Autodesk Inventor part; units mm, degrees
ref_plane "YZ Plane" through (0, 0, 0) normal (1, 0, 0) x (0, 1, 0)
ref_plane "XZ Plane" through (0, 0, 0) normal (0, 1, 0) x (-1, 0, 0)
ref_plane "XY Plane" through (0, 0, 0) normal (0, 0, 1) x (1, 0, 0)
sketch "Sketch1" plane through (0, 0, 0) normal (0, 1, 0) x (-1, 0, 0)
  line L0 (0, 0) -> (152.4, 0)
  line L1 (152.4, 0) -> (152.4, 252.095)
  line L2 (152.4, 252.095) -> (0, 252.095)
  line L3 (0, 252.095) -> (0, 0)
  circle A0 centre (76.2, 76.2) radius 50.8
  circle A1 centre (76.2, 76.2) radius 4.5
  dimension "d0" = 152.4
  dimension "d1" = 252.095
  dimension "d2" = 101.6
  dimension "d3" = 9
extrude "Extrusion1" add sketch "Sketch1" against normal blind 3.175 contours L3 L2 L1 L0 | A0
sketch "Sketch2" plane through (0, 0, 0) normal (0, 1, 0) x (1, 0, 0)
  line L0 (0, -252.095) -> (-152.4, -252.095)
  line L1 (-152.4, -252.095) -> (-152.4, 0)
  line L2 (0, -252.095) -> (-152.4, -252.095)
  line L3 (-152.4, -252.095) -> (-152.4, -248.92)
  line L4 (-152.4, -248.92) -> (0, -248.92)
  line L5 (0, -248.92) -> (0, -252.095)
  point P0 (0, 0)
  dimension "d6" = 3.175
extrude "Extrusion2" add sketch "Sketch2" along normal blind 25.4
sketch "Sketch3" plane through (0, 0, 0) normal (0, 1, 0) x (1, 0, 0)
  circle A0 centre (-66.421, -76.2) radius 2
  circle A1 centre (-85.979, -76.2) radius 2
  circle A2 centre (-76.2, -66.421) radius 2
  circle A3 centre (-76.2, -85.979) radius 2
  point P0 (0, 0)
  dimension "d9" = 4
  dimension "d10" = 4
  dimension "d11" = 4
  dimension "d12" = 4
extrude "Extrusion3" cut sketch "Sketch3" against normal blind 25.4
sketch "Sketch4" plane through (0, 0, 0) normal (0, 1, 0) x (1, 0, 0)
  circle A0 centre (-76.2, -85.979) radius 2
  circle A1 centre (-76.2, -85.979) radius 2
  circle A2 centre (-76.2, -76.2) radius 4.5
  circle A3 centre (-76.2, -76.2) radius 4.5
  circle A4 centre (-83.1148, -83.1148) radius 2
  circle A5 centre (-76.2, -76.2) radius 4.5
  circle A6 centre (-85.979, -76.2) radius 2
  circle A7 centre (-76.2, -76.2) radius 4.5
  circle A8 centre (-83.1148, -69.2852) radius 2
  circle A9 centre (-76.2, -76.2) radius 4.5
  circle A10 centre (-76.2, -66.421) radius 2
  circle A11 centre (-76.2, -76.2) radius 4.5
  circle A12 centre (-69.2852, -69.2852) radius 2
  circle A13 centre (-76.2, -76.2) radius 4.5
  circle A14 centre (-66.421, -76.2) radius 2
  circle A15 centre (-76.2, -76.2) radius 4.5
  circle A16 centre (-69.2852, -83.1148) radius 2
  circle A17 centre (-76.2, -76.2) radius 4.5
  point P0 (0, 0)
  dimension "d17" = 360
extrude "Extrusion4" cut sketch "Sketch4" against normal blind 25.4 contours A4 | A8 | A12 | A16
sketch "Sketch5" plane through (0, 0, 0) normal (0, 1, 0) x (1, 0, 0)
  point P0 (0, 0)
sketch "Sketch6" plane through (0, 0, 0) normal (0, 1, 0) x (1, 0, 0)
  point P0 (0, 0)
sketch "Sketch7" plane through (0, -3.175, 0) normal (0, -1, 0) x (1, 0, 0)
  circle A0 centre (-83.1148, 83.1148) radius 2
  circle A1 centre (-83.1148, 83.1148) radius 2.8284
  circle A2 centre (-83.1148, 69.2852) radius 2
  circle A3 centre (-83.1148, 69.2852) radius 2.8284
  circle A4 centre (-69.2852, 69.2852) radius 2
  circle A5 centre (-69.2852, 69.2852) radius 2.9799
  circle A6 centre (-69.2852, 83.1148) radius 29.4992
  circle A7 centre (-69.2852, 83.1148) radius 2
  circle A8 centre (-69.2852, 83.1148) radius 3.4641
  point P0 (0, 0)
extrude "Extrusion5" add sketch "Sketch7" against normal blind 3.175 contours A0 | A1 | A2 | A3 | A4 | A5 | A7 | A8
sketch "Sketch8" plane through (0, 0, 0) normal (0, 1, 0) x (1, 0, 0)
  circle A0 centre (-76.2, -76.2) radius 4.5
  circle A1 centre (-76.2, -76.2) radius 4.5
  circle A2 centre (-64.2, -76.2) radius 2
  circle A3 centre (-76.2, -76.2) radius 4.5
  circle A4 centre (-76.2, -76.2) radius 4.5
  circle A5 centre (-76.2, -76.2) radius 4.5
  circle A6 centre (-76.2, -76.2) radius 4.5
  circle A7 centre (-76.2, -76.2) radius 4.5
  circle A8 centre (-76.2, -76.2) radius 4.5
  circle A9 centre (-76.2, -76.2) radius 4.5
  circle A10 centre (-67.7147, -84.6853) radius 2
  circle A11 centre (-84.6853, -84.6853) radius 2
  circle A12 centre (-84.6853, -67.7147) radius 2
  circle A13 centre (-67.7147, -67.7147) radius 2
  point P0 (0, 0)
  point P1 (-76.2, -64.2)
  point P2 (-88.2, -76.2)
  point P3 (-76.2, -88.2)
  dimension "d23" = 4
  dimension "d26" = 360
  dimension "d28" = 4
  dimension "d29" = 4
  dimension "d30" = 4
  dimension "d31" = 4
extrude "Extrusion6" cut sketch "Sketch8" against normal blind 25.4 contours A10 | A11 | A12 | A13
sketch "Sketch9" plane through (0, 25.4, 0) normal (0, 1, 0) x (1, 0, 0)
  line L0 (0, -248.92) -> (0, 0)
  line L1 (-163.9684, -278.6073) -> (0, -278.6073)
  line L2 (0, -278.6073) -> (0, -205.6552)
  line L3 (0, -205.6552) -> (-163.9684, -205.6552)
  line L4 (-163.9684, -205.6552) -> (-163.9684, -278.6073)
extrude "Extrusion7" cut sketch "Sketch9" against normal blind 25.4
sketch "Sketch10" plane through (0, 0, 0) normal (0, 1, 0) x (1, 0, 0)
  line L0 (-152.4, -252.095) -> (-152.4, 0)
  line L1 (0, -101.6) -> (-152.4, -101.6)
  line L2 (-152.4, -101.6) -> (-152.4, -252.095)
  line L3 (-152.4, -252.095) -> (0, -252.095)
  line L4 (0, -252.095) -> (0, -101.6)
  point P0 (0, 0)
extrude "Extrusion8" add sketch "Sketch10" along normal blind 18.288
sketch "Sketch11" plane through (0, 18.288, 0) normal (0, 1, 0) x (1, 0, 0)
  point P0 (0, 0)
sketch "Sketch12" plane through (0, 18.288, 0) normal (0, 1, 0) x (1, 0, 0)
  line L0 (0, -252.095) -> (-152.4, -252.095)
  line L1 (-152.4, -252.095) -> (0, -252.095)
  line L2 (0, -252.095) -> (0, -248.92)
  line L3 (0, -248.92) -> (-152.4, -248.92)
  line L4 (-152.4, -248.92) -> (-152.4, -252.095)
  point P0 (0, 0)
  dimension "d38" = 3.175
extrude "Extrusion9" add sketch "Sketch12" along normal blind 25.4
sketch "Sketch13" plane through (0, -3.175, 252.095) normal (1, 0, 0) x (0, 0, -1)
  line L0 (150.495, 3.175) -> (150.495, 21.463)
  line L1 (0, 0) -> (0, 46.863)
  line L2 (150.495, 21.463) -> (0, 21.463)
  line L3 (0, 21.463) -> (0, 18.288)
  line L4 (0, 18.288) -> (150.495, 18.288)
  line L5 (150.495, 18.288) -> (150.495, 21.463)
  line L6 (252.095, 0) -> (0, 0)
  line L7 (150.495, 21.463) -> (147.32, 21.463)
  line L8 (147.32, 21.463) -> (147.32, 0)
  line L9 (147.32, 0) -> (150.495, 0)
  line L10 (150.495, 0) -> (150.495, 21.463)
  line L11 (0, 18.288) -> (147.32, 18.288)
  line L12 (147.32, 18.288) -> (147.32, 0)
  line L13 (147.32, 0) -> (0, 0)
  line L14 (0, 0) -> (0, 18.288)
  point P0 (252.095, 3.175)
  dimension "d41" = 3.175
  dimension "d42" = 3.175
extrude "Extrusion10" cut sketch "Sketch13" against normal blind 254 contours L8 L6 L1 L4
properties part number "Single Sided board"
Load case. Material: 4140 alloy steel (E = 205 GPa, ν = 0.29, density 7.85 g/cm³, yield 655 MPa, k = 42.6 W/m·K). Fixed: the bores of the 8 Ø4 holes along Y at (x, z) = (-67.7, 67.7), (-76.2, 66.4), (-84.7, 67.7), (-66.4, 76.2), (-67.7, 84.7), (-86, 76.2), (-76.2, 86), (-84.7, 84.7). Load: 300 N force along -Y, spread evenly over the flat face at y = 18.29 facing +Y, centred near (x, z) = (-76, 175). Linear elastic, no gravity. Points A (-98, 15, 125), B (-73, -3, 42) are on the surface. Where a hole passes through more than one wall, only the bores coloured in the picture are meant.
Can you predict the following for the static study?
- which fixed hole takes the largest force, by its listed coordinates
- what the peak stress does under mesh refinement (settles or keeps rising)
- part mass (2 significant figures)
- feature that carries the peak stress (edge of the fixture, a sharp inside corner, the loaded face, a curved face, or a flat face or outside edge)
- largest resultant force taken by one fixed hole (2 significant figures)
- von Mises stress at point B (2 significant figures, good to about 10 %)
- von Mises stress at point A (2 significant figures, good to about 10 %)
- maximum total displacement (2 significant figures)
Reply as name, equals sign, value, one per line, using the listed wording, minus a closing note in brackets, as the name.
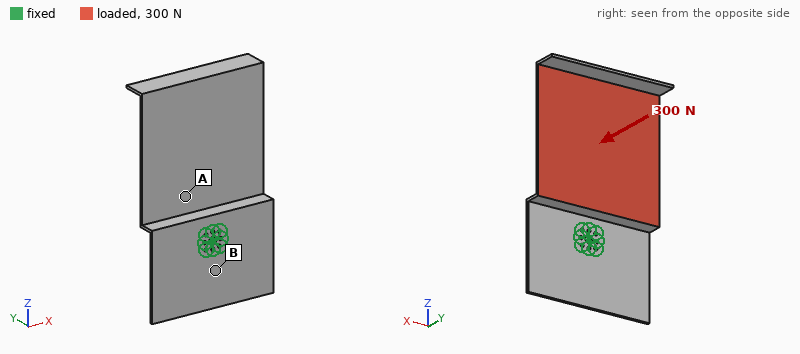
which fixed hole takes the largest force, by its listed coordinates = (-76.2, 86)
what the peak stress does under mesh refinement = keeps rising
part mass = 1.1 kg
feature that carries the peak stress = edge of the fixture
largest resultant force taken by one fixed hole = 430 N
von Mises stress at point B = 21 MPa
von Mises stress at point A = 55 MPa
maximum total displacement = 3.1 mm
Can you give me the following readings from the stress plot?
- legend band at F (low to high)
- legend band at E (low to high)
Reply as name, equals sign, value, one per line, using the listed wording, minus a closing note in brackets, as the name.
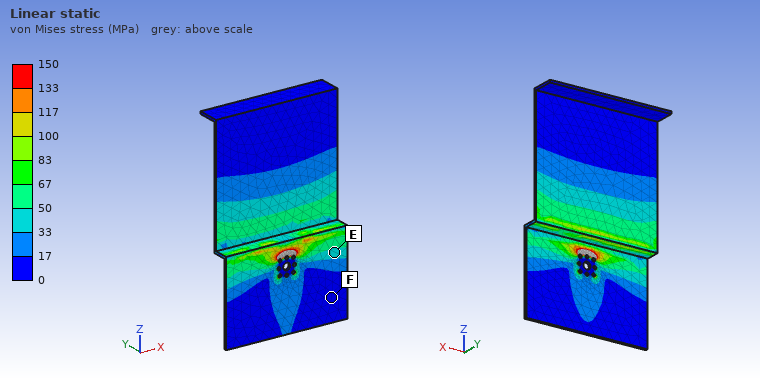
legend band at F = 0 to 17 MPa
legend band at E = 33 to 50 MPa
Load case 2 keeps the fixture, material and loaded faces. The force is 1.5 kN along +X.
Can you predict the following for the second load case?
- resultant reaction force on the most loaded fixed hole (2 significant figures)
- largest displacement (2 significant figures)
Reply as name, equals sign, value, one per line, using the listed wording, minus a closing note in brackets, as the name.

resultant reaction force on the most loaded fixed hole = 2.2 kN
largest displacement = 0.49 mm
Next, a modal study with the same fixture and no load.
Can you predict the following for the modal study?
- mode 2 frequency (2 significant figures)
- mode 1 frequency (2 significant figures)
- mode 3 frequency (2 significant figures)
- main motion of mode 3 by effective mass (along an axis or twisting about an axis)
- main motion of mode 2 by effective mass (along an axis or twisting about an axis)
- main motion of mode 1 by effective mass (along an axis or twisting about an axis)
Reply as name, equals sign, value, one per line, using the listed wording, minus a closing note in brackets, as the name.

mode 2 frequency = 180 Hz
mode 1 frequency = 64 Hz
mode 3 frequency = 360 Hz
main motion of mode 3 by effective mass = along X
main motion of mode 2 by effective mass = twisting about Z
main motion of mode 1 by effective mass = along Y
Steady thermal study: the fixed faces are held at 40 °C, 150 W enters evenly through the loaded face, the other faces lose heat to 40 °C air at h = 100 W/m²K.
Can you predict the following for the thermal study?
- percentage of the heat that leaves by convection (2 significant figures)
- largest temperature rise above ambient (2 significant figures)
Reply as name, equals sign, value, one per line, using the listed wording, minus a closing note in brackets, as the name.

percentage of the heat that leaves by convection = 97 %
largest temperature rise above ambient = 56 K
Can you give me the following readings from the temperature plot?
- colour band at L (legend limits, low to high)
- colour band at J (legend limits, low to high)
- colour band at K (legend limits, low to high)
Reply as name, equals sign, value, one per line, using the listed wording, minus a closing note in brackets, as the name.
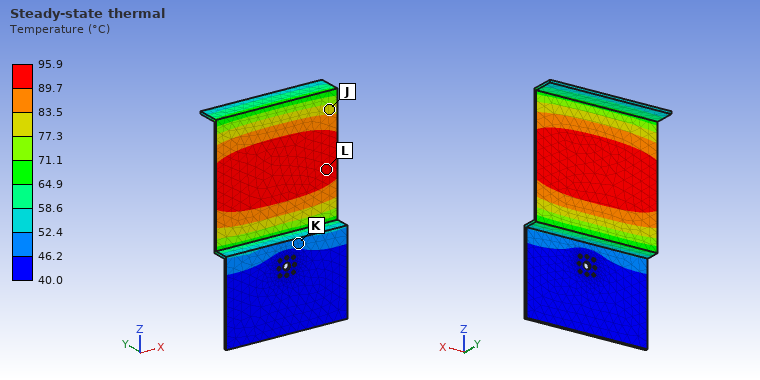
colour band at L = 89.7 to 95.9 °C
colour band at J = 77.3 to 83.5 °C
colour band at K = 46.2 to 52.4 °C
